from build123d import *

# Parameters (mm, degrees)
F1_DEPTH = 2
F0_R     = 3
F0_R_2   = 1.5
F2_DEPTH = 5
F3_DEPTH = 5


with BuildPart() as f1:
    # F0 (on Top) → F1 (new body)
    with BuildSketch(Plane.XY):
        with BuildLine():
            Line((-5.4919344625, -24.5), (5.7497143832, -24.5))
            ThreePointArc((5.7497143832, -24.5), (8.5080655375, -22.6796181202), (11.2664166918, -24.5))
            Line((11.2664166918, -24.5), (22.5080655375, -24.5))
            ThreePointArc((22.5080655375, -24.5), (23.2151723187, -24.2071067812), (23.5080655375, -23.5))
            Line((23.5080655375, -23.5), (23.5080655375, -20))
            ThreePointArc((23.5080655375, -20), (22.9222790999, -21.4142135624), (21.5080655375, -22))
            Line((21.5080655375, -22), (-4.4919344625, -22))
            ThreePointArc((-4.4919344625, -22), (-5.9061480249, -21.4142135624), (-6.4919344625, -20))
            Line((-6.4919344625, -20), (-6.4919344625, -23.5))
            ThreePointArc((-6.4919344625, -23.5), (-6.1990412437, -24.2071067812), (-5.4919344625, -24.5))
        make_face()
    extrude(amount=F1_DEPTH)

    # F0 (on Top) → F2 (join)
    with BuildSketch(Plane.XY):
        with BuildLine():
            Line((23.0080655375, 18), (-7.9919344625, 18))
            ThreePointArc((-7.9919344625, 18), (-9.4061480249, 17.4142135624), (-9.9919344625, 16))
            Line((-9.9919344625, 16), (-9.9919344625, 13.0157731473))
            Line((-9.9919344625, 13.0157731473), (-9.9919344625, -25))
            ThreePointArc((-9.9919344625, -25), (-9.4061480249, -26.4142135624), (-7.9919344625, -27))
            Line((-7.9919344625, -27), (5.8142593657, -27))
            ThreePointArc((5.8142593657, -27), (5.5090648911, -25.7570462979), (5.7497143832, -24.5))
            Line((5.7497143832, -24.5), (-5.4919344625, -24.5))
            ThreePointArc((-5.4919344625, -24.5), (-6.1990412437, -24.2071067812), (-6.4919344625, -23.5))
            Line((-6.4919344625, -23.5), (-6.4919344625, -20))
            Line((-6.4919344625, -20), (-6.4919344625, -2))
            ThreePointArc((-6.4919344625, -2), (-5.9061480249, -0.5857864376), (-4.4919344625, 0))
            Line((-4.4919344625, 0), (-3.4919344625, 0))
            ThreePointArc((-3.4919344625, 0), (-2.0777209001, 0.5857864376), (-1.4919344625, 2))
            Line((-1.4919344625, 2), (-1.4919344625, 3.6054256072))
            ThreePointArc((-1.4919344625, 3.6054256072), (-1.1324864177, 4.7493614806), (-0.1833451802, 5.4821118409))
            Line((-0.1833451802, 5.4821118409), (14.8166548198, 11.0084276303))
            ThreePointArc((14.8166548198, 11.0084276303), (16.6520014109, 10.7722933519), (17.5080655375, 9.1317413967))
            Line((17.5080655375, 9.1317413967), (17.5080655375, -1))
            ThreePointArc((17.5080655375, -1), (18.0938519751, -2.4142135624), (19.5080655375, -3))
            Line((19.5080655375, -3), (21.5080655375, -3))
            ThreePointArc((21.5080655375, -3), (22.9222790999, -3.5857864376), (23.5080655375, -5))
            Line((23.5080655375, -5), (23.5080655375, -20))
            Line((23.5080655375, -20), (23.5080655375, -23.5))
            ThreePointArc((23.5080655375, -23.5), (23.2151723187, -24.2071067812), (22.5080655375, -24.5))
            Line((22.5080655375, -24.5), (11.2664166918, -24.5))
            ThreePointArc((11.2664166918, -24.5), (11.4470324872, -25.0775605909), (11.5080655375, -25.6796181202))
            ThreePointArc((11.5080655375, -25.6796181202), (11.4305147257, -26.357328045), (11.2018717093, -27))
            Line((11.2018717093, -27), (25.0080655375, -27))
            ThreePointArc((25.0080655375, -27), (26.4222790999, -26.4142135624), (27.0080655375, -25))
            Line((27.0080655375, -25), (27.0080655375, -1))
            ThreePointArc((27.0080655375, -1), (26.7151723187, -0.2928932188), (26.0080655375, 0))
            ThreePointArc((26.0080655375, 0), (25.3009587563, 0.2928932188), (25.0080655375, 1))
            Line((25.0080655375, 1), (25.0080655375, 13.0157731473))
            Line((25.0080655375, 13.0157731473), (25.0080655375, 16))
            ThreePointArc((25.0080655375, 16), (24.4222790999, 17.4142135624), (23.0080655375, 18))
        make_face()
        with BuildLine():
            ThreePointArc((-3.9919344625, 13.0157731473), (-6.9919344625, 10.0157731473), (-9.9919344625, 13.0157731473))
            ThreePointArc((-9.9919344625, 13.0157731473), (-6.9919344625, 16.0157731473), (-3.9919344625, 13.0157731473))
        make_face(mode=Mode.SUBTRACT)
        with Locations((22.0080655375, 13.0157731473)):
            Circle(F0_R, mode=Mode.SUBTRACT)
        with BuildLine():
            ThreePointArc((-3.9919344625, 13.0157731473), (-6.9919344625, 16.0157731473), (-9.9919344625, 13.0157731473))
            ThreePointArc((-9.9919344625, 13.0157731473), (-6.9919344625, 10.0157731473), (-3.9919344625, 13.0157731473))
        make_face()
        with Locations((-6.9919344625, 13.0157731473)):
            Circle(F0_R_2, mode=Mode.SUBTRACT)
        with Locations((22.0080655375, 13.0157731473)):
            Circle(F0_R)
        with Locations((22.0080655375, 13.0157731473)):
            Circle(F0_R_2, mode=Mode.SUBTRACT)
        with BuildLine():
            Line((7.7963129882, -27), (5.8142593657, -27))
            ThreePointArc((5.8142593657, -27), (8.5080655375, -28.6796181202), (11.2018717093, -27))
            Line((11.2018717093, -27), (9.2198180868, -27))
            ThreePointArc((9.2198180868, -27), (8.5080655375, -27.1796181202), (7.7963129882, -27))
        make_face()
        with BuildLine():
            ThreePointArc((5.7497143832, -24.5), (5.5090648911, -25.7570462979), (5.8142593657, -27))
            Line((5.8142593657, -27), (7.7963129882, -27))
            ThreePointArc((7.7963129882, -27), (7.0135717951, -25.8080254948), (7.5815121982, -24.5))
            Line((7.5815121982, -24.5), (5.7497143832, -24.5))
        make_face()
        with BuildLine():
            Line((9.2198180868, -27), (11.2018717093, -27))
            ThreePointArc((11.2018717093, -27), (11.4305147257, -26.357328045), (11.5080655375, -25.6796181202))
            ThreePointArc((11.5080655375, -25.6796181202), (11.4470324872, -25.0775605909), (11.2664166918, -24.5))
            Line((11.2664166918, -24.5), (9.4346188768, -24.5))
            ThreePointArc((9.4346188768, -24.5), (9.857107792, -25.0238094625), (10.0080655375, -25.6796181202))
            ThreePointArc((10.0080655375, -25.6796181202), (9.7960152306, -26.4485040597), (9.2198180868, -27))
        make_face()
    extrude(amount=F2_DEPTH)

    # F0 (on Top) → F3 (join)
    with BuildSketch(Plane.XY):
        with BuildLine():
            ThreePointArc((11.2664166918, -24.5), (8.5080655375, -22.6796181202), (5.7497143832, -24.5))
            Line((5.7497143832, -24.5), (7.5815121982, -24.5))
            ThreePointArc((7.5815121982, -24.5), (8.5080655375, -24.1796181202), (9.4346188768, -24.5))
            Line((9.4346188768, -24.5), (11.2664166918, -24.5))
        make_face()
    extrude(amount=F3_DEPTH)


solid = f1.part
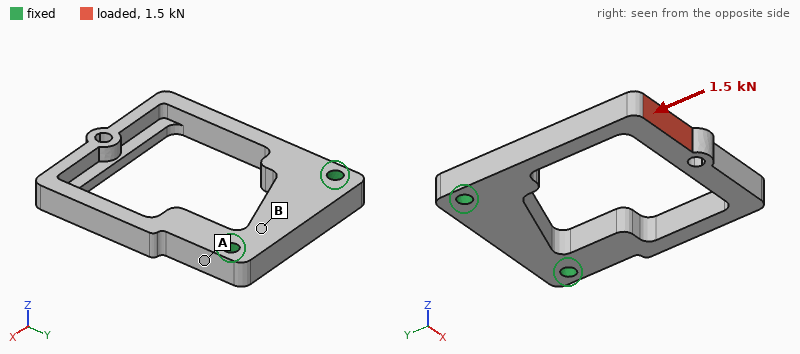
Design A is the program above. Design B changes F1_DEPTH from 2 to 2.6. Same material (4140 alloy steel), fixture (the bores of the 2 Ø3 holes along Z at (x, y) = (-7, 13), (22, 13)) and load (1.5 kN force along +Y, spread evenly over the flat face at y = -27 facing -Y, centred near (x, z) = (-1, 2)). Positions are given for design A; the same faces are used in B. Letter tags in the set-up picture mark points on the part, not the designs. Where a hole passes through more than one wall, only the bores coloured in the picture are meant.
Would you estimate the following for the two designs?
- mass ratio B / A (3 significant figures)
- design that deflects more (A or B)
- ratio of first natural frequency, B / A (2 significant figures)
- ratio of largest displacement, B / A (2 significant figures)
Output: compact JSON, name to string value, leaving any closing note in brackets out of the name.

{"mass ratio B / A": "1.01", "design that deflects more": "A", "ratio of first natural frequency, B / A": "0.98", "ratio of largest displacement, B / A": "0.89"}
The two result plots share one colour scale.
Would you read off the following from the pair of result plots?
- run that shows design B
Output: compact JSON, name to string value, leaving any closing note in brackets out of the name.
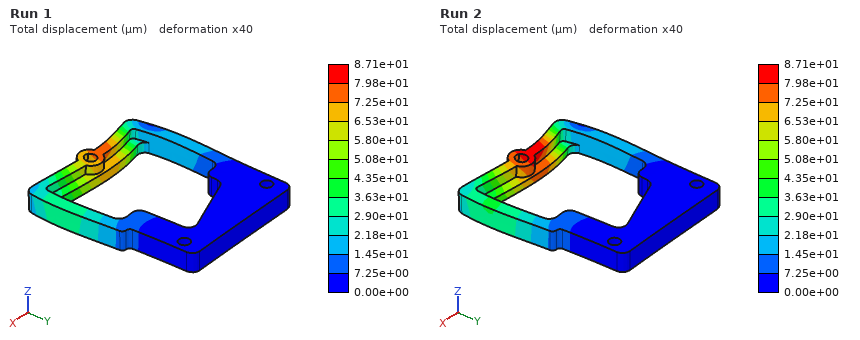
{"run that shows design B": "Run 1"}
